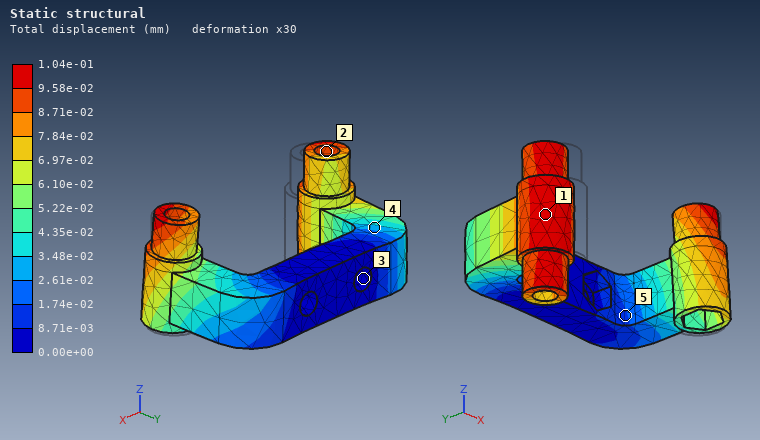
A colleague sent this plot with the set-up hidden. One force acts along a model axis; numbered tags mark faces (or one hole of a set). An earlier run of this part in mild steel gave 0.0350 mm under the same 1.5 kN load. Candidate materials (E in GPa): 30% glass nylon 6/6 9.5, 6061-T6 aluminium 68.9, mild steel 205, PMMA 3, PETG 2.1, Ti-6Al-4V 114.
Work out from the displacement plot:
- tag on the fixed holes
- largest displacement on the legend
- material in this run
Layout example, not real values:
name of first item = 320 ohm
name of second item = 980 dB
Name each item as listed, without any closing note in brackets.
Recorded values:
tag on the fixed holes = 3
largest displacement on the legend = 1.04e-01 mm
material in this run = 6061-T6 aluminium
